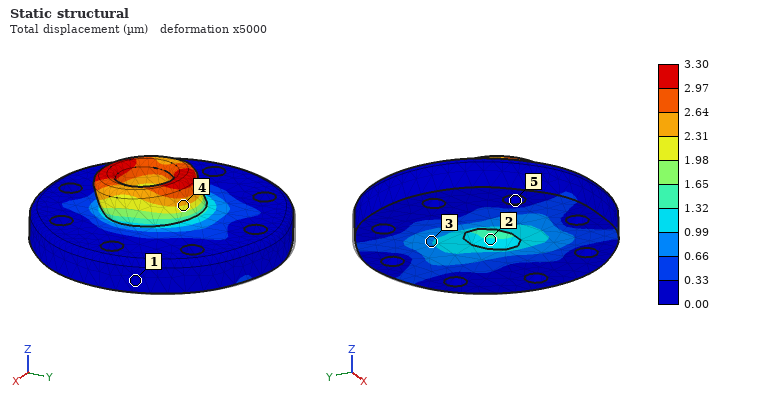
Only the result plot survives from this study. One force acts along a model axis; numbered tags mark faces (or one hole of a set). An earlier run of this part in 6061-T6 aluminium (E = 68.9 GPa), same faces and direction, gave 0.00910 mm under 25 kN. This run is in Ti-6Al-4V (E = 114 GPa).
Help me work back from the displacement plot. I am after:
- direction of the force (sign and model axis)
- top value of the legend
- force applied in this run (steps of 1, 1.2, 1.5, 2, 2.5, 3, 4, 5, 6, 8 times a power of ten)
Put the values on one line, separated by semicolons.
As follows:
-Y; 3.30 µm; 15 kN
